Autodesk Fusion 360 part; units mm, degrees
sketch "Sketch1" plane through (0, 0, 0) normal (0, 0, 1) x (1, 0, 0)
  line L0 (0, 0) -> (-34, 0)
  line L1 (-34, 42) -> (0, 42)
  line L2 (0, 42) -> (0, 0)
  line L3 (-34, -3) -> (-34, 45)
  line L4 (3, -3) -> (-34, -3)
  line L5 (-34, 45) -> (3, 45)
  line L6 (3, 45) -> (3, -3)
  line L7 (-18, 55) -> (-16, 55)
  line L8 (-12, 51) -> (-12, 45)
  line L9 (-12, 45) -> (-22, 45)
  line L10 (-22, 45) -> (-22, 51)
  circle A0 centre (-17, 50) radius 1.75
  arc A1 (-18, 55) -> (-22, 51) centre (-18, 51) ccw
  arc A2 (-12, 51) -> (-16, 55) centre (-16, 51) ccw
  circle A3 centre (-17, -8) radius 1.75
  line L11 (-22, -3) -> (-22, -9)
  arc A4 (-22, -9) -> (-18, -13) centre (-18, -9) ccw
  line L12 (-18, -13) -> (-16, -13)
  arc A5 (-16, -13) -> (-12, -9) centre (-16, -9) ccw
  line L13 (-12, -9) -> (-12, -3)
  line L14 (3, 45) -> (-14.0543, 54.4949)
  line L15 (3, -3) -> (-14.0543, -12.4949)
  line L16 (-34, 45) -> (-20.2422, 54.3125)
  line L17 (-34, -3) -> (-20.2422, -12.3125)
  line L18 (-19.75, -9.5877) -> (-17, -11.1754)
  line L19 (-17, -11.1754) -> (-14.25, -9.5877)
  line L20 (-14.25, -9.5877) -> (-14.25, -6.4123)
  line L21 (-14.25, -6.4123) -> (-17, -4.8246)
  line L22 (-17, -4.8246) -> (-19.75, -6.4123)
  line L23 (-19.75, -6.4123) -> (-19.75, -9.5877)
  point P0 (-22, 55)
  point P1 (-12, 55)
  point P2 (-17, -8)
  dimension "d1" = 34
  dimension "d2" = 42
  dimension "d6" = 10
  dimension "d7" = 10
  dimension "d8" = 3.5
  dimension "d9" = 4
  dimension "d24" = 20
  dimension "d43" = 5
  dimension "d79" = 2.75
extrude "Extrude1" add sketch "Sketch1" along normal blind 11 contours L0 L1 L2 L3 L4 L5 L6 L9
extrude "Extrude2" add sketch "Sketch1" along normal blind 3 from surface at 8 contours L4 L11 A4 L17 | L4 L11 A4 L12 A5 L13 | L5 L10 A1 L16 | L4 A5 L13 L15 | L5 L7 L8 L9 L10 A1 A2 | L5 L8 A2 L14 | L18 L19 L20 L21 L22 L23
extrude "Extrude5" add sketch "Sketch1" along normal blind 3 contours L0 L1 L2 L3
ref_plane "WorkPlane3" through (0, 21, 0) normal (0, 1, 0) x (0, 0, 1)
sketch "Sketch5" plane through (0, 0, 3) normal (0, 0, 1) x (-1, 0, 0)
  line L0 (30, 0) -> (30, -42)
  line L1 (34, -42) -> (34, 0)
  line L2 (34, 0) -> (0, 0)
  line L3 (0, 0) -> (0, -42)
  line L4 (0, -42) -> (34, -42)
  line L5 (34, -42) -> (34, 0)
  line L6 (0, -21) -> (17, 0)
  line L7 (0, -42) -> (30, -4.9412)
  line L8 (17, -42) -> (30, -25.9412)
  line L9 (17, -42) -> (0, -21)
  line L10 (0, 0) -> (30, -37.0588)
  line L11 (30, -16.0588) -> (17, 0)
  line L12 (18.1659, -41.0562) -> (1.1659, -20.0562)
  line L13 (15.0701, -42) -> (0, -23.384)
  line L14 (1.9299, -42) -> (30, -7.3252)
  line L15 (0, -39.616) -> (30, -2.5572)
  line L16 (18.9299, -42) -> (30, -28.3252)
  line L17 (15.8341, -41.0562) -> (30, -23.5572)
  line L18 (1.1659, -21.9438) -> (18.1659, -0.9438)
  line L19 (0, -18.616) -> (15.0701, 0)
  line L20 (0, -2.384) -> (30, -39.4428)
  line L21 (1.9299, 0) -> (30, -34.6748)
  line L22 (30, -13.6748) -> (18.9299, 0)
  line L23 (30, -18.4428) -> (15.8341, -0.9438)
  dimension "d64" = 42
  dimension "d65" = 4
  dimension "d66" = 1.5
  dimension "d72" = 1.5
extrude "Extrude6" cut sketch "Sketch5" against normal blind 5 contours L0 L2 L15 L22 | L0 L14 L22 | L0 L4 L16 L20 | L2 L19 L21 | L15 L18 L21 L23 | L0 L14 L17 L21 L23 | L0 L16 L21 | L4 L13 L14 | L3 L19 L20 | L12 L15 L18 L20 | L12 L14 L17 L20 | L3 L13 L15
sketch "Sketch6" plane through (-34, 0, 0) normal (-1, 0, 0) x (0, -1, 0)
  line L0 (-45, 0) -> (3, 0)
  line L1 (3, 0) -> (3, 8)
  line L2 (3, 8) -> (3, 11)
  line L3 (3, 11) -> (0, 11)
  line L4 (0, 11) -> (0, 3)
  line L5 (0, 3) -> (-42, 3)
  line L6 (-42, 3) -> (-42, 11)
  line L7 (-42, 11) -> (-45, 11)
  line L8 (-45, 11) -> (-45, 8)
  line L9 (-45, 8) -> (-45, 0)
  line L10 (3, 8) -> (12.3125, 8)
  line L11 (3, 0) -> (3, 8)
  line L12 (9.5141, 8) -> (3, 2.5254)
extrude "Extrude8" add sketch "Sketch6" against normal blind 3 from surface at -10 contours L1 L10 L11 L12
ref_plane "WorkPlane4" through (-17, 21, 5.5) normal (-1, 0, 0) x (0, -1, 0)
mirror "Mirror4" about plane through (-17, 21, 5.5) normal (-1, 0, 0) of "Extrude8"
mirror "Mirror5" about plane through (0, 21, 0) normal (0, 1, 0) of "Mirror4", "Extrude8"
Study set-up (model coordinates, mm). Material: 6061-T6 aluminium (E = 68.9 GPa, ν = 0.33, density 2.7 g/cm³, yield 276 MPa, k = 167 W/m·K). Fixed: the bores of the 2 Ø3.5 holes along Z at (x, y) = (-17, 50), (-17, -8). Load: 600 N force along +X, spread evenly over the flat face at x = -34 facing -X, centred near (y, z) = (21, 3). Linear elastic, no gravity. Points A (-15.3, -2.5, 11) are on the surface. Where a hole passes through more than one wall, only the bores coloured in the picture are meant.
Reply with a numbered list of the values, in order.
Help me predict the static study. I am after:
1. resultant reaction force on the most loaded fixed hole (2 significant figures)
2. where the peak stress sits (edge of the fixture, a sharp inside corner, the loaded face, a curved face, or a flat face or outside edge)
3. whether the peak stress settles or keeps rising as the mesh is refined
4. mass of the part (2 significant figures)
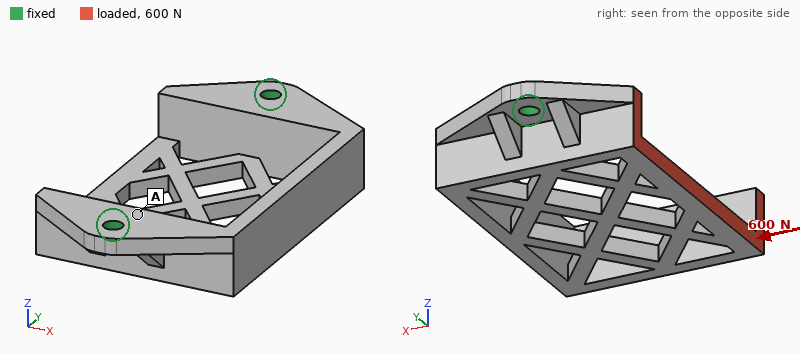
1. 300 N
2. edge of the fixture
3. keeps rising
4. 20 g
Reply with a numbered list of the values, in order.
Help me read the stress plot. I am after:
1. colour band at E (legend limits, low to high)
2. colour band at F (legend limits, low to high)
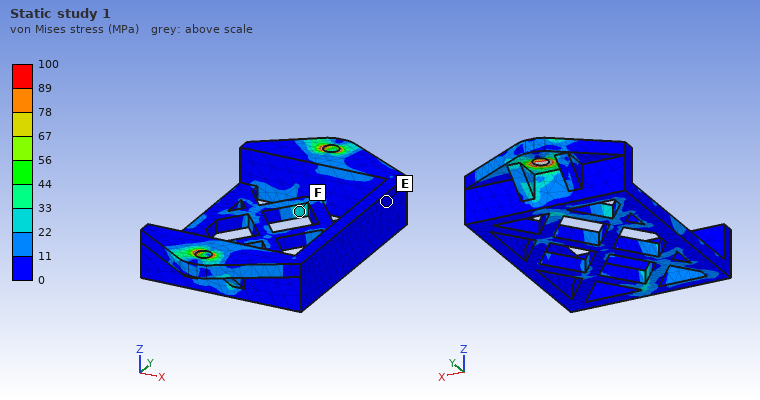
1. 0 to 11 MPa
2. 22 to 33 MPa
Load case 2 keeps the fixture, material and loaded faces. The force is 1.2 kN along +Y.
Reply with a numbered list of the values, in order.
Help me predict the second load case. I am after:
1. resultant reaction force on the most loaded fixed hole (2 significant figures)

1. 690 N
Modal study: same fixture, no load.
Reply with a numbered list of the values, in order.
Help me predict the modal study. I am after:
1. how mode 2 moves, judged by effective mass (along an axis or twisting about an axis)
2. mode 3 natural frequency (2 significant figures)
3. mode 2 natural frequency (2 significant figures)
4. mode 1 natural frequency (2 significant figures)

1. along Z
2. 6600 Hz
3. 5800 Hz
4. 3600 Hz
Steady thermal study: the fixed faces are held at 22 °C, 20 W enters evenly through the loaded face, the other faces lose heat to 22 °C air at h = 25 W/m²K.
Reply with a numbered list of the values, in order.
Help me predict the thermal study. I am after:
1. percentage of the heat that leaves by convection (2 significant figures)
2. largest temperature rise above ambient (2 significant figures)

1. 8.6 %
2. 36 K
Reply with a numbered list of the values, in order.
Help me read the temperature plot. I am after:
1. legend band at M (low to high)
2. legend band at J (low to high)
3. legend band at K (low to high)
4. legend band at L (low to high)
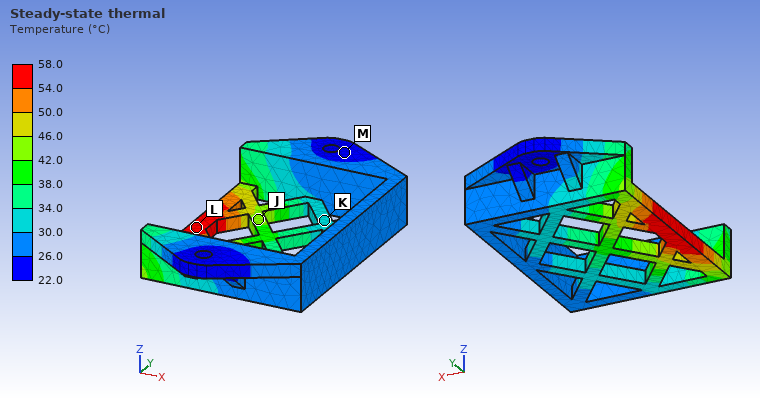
1. 22.0 to 26.0 °C
2. 42.0 to 46.0 °C
3. 30.0 to 34.0 °C
4. 54.0 to 58.0 °C
